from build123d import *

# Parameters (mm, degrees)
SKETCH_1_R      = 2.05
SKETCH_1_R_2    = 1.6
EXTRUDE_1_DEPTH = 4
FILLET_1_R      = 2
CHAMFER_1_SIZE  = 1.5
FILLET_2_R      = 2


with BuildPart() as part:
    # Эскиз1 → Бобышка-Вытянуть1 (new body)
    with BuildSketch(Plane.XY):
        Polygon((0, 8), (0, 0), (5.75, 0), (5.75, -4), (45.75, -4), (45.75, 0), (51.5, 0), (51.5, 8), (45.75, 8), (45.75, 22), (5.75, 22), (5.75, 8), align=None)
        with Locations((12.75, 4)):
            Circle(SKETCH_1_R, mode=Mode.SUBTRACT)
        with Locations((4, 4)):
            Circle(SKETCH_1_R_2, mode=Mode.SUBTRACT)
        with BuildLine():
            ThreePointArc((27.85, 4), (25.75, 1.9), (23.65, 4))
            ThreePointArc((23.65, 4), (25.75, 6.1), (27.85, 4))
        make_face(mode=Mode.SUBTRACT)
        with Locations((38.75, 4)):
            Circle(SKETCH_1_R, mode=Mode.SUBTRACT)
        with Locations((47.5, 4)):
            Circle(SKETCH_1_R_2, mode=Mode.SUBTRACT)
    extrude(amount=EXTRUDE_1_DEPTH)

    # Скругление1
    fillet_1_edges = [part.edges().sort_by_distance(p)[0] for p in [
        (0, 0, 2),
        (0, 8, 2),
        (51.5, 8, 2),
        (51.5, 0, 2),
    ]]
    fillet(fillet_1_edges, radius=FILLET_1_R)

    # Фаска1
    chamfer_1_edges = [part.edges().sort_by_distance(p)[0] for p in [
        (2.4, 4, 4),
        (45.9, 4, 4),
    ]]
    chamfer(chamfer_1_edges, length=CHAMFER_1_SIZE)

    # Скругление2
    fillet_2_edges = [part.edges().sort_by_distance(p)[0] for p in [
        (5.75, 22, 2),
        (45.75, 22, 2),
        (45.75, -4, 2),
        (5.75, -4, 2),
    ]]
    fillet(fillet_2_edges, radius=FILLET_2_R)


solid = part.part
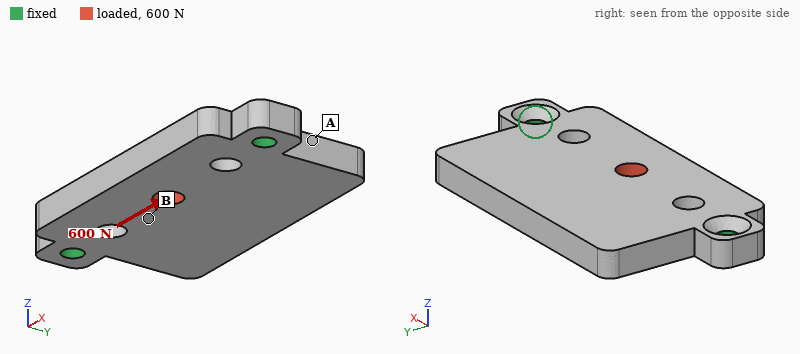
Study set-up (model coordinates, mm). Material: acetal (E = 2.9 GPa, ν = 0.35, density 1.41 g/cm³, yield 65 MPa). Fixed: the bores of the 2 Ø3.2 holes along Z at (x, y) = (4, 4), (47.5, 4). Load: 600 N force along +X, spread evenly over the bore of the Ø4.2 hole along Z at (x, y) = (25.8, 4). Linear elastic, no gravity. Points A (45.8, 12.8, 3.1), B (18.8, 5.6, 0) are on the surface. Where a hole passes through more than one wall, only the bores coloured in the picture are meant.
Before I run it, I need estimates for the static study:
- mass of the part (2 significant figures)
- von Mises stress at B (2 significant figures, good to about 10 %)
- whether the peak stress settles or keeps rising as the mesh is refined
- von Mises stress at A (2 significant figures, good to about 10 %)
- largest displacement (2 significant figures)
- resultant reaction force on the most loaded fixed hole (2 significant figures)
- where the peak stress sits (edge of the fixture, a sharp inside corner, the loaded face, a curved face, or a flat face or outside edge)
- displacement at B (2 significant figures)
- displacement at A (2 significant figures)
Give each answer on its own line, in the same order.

6.0 g
7.4 MPa
keeps rising
2.8 MPa
70 µm
300 N
edge of the fixture
53 µm
37 µm
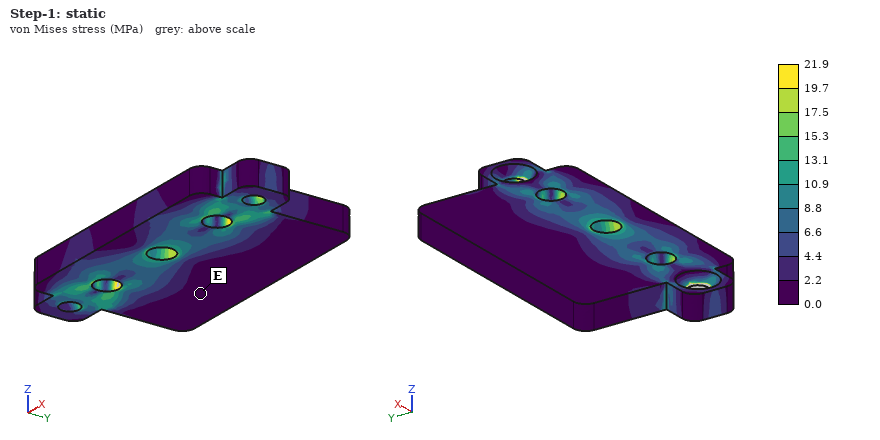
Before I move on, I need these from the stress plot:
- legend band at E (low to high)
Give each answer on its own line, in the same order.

0.0 to 2.2 MPa
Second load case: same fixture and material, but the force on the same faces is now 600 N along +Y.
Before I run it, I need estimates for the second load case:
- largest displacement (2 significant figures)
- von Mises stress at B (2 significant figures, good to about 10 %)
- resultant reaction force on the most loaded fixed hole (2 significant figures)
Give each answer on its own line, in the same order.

0.18 mm
7.1 MPa
310 N
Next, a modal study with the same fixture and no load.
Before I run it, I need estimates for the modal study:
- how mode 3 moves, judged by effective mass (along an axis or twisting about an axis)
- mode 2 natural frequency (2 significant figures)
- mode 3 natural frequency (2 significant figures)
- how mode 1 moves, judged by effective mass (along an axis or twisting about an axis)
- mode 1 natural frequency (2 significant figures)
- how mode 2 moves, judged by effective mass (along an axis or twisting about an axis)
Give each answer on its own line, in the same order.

twisting about Y
2500 Hz
3200 Hz
along Z
1300 Hz
along Z
